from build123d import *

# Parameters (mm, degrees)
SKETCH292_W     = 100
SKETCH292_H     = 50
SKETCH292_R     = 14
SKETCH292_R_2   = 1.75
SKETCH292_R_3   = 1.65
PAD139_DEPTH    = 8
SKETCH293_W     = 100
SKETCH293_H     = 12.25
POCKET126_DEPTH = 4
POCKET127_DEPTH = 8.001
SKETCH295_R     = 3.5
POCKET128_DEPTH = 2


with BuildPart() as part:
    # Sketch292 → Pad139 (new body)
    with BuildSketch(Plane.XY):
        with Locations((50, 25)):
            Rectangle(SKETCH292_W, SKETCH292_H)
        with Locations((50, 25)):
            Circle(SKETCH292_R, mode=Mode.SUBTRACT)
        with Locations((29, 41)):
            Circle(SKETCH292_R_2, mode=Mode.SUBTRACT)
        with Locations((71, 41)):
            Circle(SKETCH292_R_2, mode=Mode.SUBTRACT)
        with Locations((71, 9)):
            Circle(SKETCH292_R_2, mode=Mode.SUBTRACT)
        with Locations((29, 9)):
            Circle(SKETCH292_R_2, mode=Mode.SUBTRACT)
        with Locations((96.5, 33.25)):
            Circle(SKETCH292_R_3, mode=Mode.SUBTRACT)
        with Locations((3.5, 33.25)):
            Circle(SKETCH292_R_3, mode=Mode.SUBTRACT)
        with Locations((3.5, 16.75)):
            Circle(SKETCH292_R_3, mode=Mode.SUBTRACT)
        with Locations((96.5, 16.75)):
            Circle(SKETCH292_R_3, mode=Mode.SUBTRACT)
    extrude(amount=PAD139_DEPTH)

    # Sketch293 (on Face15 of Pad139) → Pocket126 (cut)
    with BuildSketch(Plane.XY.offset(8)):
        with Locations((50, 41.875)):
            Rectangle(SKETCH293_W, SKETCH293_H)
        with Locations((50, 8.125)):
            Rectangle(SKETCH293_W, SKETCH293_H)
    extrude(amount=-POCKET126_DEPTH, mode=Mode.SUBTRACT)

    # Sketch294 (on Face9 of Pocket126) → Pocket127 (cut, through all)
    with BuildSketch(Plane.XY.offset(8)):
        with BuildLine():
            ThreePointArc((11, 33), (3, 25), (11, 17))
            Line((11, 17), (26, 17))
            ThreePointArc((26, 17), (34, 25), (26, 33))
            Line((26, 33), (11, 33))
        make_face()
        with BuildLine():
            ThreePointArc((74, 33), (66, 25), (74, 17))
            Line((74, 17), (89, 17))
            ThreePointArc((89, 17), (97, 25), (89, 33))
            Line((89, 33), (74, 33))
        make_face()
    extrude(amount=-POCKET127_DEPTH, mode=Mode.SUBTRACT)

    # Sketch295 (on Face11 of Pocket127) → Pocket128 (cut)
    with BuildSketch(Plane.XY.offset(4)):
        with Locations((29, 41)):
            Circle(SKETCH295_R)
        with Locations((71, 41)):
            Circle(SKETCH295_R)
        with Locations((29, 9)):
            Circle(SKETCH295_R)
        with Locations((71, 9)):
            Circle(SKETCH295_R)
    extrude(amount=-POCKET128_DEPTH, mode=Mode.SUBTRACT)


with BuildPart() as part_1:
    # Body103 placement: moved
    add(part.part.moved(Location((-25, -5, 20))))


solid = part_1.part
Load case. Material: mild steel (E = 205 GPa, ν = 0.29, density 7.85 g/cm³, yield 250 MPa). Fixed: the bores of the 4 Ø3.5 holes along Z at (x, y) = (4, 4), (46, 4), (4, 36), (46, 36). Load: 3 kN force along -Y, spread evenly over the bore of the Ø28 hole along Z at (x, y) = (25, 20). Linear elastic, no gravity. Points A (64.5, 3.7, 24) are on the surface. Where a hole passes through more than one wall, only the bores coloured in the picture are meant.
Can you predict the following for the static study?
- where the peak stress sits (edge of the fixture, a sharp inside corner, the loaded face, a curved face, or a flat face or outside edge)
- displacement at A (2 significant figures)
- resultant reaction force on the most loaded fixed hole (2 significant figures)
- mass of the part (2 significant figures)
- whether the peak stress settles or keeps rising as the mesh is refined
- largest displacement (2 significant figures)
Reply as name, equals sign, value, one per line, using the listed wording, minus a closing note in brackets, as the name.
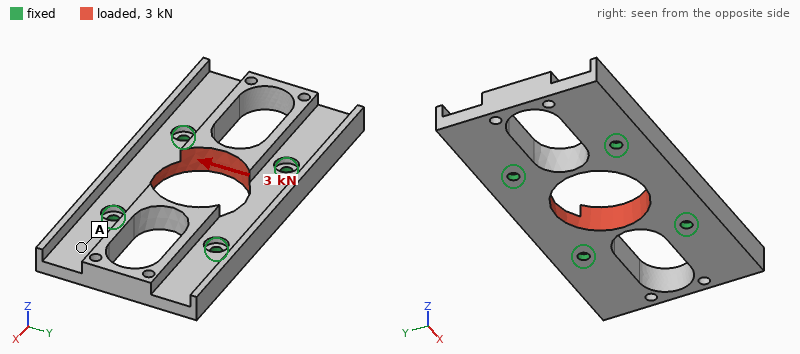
where the peak stress sits = edge of the fixture
displacement at A = 1.5 µm
resultant reaction force on the most loaded fixed hole = 760 N
mass of the part = 140 g
whether the peak stress settles or keeps rising as the mesh is refined = keeps rising
largest displacement = 5.8 µm
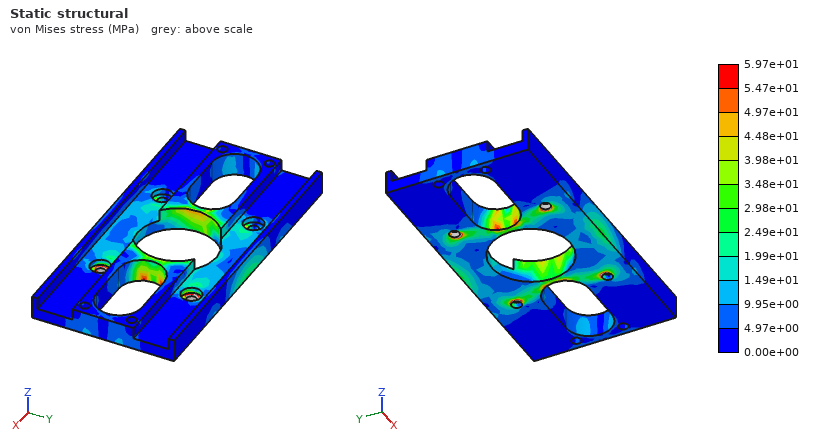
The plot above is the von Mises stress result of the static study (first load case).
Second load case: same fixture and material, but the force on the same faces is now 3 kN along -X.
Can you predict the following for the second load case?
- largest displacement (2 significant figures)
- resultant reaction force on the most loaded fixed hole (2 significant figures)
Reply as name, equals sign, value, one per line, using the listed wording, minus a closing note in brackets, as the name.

largest displacement = 8.4 µm
resultant reaction force on the most loaded fixed hole = 770 N
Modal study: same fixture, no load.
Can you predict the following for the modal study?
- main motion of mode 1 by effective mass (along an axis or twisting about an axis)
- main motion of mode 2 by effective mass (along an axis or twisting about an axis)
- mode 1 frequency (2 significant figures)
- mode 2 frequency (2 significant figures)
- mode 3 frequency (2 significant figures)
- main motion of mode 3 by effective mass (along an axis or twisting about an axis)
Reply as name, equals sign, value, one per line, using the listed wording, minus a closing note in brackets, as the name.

main motion of mode 1 by effective mass = along Z
main motion of mode 2 by effective mass = twisting about Y
mode 1 frequency = 3500 Hz
mode 2 frequency = 3900 Hz
mode 3 frequency = 5500 Hz
main motion of mode 3 by effective mass = twisting about X
